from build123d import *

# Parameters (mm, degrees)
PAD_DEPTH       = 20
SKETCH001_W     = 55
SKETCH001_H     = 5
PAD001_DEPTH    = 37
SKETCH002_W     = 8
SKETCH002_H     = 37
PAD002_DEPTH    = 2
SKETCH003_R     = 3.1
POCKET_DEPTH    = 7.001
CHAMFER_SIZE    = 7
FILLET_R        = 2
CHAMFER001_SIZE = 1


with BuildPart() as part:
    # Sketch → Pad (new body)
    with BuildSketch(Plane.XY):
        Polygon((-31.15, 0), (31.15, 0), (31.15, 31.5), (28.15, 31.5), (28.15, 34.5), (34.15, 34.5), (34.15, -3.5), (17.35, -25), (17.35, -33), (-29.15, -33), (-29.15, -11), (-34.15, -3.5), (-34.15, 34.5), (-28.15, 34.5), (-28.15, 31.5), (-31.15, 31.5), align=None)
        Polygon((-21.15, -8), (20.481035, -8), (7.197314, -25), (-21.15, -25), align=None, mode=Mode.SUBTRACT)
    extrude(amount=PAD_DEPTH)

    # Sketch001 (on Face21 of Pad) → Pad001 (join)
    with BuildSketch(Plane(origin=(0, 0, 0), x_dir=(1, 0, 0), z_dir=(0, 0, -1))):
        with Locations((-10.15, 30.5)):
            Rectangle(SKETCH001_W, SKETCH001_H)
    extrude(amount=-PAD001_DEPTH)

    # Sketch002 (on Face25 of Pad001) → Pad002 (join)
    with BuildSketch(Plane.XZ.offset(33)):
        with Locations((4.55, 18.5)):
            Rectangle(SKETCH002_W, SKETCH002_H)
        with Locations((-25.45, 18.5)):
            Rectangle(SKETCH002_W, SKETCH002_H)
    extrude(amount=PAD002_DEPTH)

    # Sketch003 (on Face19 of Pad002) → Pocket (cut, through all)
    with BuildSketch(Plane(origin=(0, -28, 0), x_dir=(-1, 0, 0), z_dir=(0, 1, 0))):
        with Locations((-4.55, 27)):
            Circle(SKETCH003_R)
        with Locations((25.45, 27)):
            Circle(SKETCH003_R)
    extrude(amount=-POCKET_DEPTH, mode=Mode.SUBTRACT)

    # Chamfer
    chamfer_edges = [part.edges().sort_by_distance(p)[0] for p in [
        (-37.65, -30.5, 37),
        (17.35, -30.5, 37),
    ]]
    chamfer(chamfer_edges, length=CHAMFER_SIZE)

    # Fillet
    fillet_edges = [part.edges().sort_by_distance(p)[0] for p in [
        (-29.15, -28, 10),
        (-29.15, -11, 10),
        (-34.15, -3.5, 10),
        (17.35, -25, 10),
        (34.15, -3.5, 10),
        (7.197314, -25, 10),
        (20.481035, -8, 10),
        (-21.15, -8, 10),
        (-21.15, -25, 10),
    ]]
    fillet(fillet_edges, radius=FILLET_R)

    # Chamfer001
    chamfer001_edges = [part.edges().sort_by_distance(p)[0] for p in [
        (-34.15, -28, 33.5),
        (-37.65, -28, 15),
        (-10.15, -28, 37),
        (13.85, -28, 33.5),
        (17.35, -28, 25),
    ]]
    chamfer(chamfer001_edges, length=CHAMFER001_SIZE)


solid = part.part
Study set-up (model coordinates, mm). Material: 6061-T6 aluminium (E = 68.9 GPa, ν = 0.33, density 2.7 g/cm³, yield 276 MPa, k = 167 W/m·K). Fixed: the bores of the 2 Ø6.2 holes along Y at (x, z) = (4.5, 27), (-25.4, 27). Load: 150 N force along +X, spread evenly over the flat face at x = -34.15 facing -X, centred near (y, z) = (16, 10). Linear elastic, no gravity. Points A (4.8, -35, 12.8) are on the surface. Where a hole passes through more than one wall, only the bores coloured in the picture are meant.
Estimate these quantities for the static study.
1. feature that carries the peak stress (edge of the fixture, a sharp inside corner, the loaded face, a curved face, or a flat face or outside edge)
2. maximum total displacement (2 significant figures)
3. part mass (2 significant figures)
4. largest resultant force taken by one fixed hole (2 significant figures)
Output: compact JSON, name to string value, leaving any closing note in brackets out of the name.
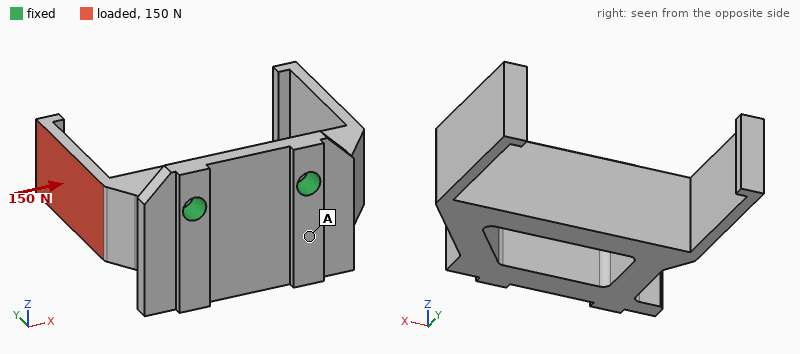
{"feature that carries the peak stress": "the loaded face", "maximum total displacement": "0.31 mm", "part mass": "94 g", "largest resultant force taken by one fixed hole": "210 N"}
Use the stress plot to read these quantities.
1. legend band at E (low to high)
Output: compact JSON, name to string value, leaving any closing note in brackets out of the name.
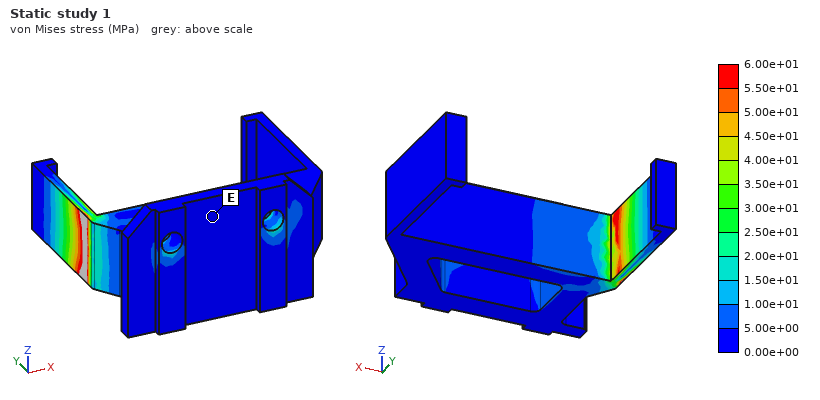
{"legend band at E": "0.00e+00 to 5.00e+00 MPa"}
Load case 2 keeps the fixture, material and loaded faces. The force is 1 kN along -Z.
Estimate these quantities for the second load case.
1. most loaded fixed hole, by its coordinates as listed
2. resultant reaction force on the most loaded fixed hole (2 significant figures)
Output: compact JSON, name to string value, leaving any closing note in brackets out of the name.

{"most loaded fixed hole, by its coordinates as listed": "(-25.4, 27)", "resultant reaction force on the most loaded fixed hole": "1.2 kN"}
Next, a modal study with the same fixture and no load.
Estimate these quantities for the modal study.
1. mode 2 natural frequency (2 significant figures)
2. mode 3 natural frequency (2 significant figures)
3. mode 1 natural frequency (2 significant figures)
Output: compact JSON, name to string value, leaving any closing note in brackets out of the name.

{"mode 2 natural frequency": "1500 Hz", "mode 3 natural frequency": "1600 Hz", "mode 1 natural frequency": "1500 Hz"}
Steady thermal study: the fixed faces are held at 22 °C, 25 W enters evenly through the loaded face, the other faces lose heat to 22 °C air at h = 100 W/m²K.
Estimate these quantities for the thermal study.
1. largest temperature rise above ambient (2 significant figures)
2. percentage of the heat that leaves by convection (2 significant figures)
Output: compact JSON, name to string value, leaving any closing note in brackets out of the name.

{"largest temperature rise above ambient": "52 K", "percentage of the heat that leaves by convection": "45 %"}
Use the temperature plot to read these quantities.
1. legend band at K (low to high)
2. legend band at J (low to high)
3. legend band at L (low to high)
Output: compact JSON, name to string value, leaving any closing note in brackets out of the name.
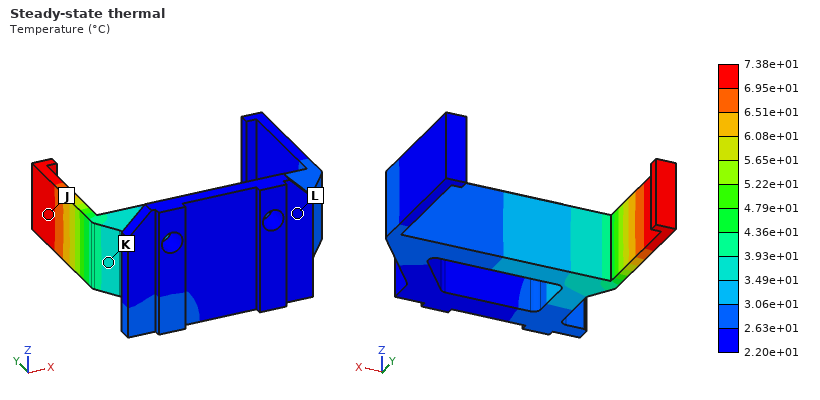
{"legend band at K": "3.49e+01 to 3.93e+01 °C", "legend band at J": "6.95e+01 to 7.38e+01 °C", "legend band at L": "2.20e+01 to 2.63e+01 °C"}
